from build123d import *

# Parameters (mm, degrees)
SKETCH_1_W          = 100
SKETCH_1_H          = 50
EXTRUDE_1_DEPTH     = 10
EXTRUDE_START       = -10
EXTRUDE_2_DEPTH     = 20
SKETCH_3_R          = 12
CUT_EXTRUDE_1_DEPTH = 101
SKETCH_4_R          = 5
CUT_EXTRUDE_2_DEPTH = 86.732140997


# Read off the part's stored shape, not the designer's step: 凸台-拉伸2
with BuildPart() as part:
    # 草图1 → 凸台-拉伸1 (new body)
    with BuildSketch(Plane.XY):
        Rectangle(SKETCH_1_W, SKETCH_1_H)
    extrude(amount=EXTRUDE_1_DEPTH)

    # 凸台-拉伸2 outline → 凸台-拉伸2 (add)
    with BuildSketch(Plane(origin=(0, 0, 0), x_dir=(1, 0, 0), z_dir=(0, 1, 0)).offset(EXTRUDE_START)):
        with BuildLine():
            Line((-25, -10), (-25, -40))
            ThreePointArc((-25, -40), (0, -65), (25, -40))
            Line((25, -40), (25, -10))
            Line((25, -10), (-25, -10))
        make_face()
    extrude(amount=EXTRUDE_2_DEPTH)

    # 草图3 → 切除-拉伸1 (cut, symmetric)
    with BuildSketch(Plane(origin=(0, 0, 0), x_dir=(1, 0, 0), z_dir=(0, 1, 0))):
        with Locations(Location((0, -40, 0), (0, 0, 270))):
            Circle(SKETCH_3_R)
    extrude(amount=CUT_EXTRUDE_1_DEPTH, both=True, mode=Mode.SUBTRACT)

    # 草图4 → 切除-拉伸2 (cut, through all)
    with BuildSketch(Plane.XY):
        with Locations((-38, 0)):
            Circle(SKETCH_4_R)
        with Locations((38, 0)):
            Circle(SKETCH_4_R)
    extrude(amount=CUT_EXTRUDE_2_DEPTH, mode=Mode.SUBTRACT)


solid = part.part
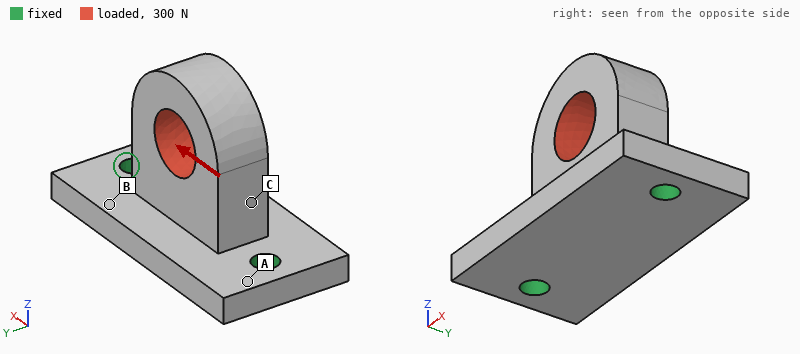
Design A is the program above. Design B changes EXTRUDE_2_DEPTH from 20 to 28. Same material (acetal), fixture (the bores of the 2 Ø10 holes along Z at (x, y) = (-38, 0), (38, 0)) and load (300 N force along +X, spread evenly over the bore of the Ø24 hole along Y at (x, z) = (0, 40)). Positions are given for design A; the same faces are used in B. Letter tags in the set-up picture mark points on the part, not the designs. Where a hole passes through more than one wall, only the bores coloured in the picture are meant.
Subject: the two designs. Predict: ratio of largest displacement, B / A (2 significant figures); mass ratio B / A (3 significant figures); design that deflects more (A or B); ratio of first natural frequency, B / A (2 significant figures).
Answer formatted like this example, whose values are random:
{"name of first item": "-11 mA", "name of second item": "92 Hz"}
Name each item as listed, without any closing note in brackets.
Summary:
{"ratio of largest displacement, B / A": "0.84", "mass ratio B / A": "1.18", "design that deflects more": "A", "ratio of first natural frequency, B / A": "0.93"}
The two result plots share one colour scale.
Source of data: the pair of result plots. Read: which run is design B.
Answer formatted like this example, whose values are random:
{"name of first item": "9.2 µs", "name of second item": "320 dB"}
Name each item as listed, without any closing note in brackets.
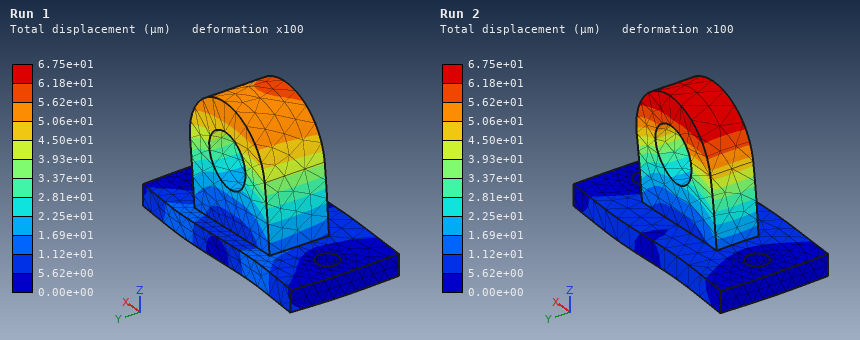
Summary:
{"which run is design B": "Run 1"}
